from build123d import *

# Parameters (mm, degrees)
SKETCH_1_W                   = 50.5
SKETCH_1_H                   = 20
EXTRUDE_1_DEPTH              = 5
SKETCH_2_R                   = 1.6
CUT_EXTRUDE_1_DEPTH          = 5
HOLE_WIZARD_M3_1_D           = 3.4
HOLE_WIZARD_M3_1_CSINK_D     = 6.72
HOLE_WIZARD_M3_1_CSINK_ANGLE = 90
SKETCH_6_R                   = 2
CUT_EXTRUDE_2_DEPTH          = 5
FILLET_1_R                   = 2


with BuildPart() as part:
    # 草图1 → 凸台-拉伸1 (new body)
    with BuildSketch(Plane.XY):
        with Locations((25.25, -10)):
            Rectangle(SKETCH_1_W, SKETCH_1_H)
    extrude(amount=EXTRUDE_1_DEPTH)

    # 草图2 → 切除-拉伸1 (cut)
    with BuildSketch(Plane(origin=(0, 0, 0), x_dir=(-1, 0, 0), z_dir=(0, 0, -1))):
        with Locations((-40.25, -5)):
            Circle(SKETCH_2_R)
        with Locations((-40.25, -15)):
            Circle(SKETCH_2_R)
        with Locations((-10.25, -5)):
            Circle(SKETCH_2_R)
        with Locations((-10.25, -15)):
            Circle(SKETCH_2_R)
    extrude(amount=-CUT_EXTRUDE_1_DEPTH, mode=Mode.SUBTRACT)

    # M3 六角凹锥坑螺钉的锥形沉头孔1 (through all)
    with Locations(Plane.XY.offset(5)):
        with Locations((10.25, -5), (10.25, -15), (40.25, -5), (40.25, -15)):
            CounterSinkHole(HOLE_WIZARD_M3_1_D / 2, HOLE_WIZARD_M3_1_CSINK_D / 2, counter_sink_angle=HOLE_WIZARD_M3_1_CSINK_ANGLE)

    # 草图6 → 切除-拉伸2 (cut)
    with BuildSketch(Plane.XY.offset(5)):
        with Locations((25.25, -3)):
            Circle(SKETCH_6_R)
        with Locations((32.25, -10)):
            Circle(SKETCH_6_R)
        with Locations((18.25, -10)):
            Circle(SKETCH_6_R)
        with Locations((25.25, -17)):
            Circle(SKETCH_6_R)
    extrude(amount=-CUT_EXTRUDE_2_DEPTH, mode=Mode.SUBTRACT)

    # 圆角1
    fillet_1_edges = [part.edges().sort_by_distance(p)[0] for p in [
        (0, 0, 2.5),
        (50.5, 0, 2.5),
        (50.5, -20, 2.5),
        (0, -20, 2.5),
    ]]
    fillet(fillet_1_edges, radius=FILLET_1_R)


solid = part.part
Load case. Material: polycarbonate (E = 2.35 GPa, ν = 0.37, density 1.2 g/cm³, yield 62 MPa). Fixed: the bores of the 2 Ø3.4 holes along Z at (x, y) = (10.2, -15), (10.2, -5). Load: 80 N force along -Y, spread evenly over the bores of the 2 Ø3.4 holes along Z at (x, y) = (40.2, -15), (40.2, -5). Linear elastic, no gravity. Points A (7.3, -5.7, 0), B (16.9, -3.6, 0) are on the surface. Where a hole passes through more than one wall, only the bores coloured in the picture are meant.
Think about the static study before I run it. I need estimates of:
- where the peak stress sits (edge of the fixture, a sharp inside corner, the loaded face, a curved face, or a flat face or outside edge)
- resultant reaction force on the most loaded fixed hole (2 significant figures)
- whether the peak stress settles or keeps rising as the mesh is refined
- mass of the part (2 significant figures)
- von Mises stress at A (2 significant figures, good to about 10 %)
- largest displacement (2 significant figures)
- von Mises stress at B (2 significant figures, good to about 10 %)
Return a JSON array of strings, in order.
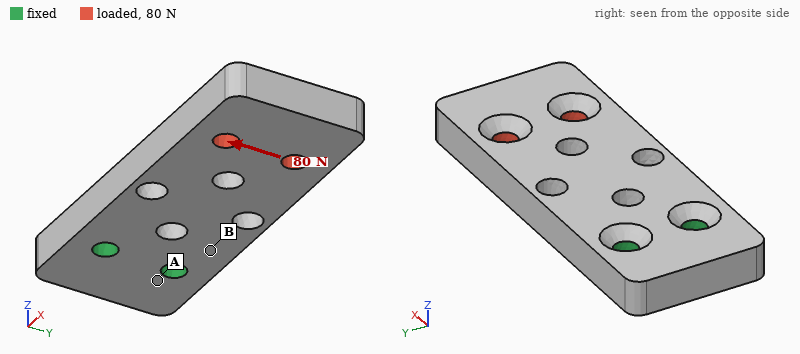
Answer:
["edge of the fixture", "200 N", "keeps rising", "5.4 g", "2.2 MPa", "0.27 mm", "5.1 MPa"]
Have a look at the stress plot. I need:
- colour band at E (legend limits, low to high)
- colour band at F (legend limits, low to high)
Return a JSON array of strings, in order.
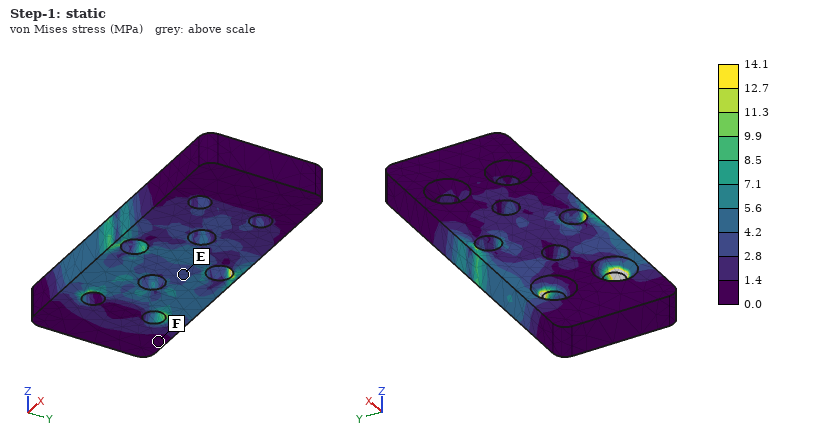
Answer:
["2.8 to 4.2 MPa", "0.0 to 1.4 MPa"]
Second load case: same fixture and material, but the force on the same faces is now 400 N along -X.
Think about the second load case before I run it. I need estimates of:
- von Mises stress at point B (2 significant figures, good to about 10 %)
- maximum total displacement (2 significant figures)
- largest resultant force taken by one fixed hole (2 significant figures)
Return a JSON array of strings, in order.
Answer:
["8.7 MPa", "0.61 mm", "200 N"]
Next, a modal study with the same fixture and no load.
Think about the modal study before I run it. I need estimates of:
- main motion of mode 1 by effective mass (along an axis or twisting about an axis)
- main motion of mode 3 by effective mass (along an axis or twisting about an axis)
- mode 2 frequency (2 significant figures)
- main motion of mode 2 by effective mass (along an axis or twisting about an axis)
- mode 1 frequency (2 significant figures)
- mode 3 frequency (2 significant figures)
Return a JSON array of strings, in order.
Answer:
["along Z", "twisting about X", "2000 Hz", "along Y", "620 Hz", "2400 Hz"]
